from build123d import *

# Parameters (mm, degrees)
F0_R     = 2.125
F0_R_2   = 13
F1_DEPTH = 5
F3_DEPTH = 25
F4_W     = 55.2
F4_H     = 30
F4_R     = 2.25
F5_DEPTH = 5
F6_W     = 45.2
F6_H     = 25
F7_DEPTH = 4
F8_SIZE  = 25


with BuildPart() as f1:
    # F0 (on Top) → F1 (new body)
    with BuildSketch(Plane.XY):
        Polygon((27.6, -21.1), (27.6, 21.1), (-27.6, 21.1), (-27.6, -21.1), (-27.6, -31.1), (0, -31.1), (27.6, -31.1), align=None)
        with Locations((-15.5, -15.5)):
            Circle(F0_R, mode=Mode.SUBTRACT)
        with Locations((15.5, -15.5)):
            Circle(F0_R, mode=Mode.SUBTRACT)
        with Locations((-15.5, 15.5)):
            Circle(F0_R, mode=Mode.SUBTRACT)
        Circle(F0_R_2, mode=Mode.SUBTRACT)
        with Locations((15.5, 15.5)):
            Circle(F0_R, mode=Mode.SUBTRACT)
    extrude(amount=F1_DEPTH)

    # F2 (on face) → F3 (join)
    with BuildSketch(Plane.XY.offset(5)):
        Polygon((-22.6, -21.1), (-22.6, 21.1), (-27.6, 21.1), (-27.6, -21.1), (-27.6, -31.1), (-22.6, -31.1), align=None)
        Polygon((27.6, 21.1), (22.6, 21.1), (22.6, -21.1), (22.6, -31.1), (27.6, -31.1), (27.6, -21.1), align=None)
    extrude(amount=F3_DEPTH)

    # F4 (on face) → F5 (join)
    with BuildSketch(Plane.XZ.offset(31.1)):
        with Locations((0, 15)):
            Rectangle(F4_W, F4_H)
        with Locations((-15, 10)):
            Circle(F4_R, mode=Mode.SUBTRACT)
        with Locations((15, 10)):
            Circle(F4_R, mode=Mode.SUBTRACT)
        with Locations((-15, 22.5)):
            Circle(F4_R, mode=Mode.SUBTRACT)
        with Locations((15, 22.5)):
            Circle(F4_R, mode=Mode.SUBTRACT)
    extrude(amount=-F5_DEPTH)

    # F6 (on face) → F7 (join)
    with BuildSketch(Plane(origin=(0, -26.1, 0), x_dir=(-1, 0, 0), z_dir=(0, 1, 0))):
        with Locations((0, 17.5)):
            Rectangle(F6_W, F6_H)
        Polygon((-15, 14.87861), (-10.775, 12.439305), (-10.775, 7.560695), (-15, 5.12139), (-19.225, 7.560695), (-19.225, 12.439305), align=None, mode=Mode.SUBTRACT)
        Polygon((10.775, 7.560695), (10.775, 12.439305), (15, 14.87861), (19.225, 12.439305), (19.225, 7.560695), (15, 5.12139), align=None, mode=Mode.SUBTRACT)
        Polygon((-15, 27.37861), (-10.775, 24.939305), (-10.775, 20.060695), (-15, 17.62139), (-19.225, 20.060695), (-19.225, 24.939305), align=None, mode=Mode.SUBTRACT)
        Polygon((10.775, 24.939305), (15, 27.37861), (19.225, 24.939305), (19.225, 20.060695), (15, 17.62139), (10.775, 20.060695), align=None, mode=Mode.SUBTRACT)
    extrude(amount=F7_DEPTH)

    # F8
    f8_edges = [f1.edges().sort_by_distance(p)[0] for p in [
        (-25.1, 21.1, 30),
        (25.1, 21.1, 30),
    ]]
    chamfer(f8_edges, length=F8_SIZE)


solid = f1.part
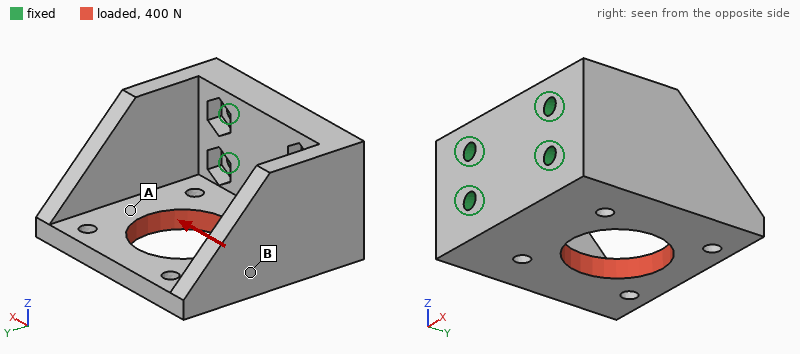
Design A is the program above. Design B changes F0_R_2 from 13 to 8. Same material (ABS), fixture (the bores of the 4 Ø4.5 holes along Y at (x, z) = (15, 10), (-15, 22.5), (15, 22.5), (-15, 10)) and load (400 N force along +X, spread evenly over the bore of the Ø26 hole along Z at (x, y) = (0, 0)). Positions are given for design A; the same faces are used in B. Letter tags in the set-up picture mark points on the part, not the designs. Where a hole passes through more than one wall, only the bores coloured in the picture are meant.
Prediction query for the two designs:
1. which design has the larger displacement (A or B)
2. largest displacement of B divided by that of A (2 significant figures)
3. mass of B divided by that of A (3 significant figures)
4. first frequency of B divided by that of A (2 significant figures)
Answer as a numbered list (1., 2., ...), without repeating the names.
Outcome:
1. A
2. 0.79
3. 1.05
4. 0.96
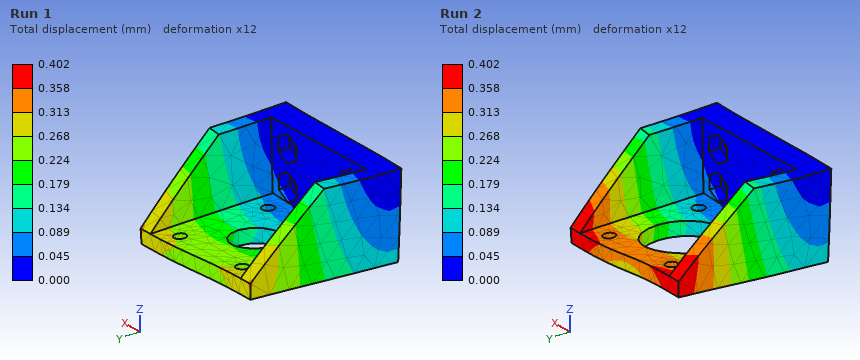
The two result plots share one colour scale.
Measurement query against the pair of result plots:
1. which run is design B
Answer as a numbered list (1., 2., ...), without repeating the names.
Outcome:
1. Run 1
